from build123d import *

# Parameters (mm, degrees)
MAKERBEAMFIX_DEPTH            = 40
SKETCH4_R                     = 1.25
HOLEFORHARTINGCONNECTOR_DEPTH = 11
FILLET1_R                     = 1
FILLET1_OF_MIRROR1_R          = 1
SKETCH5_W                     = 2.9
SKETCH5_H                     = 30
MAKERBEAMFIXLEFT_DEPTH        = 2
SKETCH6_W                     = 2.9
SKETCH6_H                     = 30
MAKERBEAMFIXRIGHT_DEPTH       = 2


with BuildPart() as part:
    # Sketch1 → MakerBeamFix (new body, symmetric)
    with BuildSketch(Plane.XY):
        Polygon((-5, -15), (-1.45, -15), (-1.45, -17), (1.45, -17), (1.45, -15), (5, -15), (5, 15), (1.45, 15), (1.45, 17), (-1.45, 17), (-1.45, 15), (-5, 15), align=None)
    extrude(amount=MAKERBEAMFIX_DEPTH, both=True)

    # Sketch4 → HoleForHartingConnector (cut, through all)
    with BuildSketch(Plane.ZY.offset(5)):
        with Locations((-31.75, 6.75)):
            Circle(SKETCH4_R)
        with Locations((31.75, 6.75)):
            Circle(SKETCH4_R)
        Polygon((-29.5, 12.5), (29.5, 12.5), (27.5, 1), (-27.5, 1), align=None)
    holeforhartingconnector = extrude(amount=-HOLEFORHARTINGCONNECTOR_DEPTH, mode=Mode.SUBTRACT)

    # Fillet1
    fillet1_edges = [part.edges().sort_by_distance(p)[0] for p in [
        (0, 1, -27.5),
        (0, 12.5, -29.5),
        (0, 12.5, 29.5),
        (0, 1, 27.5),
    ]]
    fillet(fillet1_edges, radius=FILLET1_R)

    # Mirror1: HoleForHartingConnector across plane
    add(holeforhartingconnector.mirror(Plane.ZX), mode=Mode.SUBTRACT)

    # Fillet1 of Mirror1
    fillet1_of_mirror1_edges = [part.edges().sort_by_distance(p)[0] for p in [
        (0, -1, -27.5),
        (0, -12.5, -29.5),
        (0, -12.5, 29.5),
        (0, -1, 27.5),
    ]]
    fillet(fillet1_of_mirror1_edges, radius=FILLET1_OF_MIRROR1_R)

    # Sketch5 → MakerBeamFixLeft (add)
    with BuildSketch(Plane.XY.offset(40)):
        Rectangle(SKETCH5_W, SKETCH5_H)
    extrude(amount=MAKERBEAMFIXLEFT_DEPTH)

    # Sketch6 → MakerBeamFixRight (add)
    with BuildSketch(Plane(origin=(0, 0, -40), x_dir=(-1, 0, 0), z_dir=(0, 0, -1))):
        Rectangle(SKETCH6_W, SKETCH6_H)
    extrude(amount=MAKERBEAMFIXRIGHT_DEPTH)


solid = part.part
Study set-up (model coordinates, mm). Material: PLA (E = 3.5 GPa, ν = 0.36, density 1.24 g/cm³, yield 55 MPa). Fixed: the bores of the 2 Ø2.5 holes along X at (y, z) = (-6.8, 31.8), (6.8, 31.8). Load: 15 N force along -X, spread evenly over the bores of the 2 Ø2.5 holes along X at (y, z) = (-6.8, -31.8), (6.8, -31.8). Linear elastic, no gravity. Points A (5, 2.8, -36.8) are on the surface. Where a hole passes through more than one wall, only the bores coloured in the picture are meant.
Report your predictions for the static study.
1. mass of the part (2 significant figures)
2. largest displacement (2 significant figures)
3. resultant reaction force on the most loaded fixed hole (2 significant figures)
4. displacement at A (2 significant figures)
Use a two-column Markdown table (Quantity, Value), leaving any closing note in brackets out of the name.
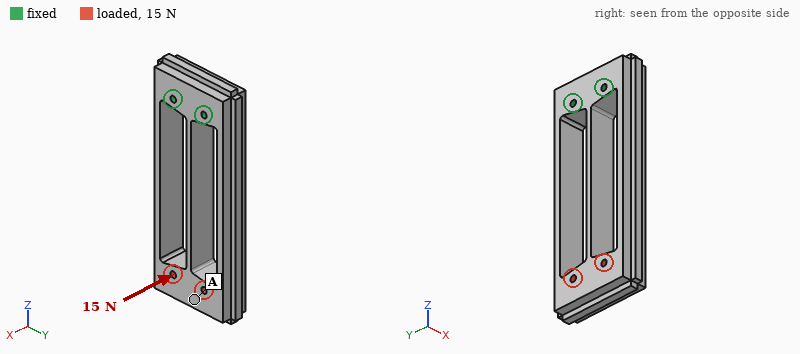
| Quantity | Value |
|---|---|
| mass of the part | 15 g |
| largest displacement | 0.84 mm |
| resultant reaction force on the most loaded fixed hole | 7.5 N |
| displacement at A | 0.76 mm |
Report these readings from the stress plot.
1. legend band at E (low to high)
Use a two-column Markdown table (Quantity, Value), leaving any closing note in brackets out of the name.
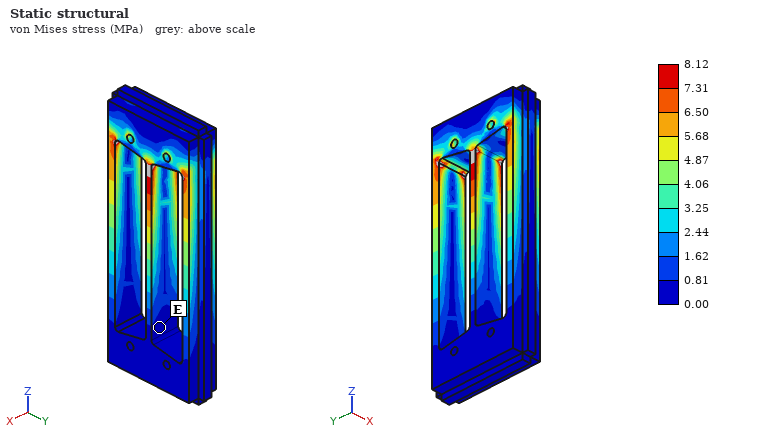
| Quantity | Value |
|---|---|
| legend band at E | 0.00 to 0.81 MPa |
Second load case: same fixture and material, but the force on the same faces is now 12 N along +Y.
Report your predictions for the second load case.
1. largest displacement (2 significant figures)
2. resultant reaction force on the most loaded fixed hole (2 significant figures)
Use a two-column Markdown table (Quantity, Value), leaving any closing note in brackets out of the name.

| Quantity | Value |
|---|---|
| largest displacement | 0.87 mm |
| resultant reaction force on the most loaded fixed hole | 46 N |
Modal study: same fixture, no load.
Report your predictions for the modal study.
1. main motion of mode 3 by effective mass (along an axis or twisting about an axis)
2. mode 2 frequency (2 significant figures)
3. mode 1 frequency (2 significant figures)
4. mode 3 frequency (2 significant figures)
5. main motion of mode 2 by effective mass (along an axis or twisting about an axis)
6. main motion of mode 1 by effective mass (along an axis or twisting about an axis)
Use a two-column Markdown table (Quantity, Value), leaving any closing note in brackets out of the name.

| Quantity | Value |
|---|---|
| main motion of mode 3 by effective mass | twisting about Z |
| mode 2 frequency | 290 Hz |
| mode 1 frequency | 230 Hz |
| mode 3 frequency | 690 Hz |
| main motion of mode 2 by effective mass | along X |
| main motion of mode 1 by effective mass | along Y |
